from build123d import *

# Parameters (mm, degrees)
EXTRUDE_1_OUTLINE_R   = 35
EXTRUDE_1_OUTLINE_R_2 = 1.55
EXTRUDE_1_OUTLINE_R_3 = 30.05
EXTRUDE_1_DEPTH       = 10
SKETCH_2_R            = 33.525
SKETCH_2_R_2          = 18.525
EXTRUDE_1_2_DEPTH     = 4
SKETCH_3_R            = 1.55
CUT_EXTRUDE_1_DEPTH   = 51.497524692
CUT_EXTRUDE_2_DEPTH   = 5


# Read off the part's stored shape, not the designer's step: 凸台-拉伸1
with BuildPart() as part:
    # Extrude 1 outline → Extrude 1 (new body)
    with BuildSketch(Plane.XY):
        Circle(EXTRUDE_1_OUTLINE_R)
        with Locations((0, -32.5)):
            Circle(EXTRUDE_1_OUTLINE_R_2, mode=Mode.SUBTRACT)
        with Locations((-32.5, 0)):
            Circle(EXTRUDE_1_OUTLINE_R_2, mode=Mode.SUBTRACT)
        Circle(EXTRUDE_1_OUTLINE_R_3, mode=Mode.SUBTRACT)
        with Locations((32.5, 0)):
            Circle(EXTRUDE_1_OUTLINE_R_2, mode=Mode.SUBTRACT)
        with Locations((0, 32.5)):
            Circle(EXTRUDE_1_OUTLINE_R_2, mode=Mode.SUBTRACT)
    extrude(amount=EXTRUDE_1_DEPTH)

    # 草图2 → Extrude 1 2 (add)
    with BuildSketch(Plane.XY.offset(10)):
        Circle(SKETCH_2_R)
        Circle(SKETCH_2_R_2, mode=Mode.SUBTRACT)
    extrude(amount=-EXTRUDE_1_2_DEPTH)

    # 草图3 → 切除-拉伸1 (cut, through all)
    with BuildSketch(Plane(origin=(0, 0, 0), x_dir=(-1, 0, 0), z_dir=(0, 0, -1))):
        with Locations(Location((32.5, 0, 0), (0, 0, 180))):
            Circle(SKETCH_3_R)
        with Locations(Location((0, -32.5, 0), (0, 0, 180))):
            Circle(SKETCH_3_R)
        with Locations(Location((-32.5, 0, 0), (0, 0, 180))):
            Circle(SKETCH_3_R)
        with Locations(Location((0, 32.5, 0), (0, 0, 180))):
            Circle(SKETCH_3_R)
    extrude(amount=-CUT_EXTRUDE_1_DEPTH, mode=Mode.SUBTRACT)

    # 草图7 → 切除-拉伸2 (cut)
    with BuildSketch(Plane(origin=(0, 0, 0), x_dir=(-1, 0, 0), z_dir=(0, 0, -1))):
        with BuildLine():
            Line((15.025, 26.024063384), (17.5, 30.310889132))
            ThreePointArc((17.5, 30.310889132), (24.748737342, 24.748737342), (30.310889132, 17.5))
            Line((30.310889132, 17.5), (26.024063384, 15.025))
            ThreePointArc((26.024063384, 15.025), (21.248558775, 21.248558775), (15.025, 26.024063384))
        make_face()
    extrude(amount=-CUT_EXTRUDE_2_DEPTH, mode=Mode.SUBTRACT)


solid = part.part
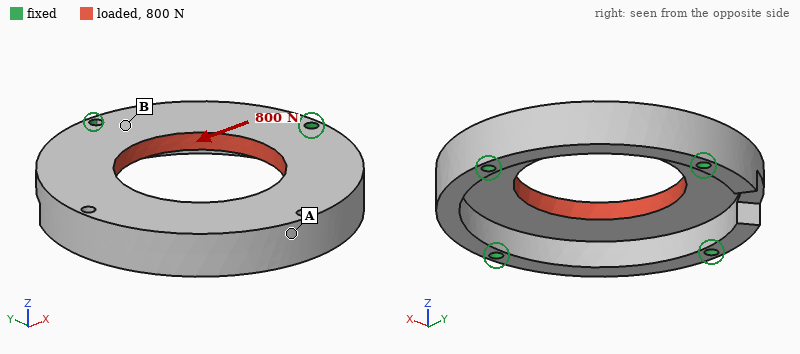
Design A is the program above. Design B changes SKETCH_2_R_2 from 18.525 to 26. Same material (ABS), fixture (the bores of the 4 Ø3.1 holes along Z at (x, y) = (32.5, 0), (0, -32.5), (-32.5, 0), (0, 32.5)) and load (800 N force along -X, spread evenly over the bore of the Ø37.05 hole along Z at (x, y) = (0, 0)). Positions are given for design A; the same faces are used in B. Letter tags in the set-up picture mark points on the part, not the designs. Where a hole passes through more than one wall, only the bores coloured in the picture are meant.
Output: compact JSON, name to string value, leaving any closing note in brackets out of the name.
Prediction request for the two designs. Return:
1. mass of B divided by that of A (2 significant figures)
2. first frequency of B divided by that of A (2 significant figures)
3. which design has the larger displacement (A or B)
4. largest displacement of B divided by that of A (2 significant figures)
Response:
{"mass of B divided by that of A": "0.75", "first frequency of B divided by that of A": "1.1", "which design has the larger displacement": "B", "largest displacement of B divided by that of A": "1.4"}
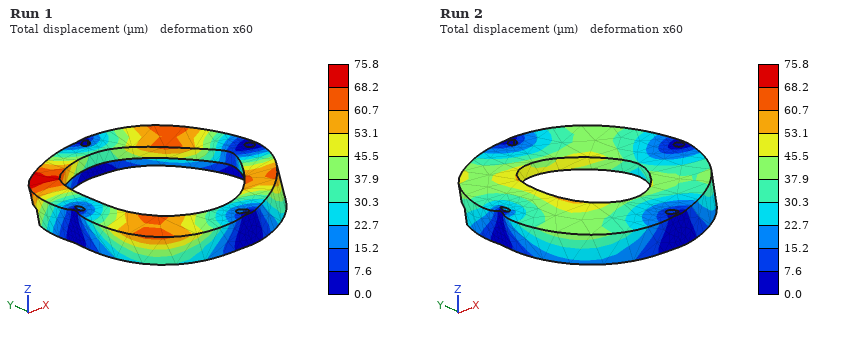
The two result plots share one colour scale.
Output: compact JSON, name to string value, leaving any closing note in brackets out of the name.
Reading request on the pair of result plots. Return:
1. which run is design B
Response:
{"which run is design B": "Run 1"}
